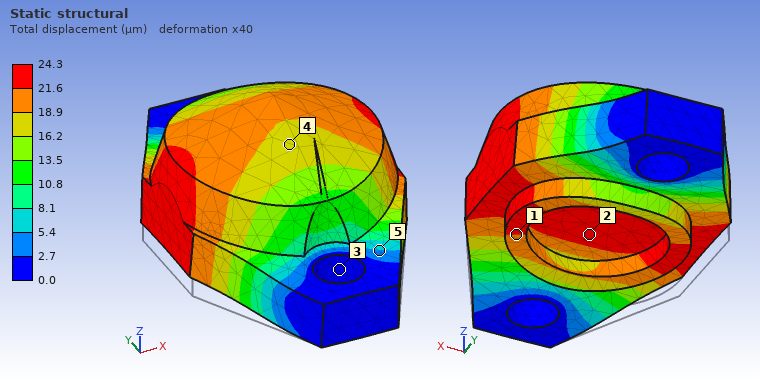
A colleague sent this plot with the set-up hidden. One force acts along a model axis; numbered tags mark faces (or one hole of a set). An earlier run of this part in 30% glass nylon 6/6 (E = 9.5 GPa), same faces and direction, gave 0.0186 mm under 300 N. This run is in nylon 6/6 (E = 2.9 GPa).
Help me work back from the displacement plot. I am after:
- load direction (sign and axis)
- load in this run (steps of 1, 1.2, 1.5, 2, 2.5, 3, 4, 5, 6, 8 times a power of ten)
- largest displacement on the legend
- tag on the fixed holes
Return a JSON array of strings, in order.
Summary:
["+Z", "120 N", "24.3 µm", "3"]
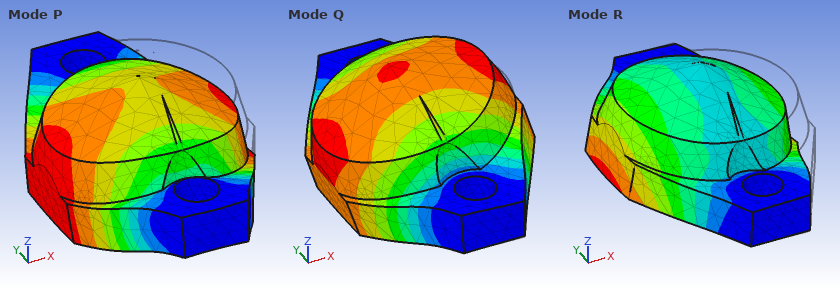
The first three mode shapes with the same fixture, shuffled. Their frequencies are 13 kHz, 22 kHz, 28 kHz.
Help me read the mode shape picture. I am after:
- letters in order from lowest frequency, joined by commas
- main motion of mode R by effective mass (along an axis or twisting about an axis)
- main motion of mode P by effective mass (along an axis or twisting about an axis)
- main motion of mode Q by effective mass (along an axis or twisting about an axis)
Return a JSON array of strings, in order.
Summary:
["Q, P, R", "along X", "along Z", "along X"]
